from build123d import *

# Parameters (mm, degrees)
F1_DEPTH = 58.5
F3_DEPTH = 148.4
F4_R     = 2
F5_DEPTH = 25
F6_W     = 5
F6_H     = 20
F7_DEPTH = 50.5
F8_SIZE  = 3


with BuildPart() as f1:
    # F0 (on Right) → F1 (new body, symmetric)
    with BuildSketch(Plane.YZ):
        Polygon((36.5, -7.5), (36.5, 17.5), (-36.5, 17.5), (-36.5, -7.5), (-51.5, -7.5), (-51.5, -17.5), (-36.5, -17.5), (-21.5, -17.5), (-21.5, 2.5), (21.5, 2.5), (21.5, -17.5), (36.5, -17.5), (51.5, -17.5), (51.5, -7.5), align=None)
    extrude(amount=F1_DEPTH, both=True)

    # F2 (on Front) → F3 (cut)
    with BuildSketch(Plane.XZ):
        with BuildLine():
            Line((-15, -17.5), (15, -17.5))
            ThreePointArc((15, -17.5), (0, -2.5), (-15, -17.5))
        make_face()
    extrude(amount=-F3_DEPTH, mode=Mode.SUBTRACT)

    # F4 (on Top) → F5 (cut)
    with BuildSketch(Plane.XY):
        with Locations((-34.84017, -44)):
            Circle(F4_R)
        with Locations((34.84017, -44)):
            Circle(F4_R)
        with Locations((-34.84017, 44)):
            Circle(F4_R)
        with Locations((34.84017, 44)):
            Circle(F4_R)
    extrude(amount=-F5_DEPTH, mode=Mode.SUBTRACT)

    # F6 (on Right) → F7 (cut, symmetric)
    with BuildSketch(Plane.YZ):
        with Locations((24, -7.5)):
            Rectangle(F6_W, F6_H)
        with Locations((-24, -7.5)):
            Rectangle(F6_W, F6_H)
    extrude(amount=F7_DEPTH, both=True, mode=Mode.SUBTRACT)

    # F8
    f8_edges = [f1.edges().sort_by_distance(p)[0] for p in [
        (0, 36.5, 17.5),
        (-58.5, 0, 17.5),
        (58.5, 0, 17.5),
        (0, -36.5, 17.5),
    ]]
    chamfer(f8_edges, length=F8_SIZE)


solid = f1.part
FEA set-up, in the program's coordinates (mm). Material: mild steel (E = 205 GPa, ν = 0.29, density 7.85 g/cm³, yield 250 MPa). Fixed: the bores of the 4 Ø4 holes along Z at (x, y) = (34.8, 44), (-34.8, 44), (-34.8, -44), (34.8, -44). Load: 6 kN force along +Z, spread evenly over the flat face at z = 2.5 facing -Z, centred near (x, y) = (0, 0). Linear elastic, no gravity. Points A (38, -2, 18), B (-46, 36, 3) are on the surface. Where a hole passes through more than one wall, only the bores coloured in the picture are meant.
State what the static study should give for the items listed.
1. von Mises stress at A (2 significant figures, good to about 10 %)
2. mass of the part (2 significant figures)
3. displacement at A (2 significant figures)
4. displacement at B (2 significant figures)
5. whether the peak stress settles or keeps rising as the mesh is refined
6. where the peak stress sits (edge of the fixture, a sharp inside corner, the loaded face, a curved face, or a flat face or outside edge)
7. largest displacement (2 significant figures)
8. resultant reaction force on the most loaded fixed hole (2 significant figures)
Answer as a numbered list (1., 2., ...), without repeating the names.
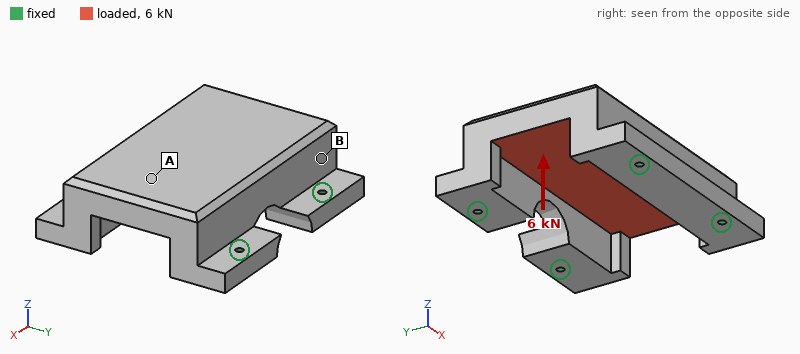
1. 6.9 MPa
2. 1.6 kg
3. 3.6 µm
4. 1.8 µm
5. keeps rising
6. edge of the fixture
7. 4.0 µm
8. 1.9 kN
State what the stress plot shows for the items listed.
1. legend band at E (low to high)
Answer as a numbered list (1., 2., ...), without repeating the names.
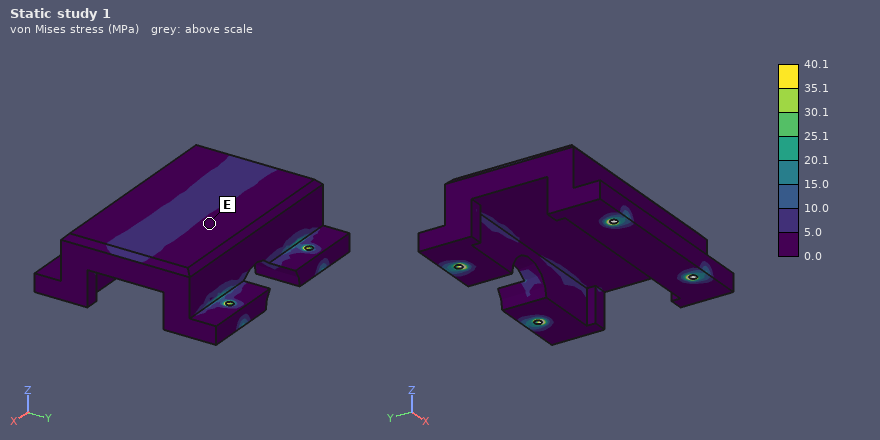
1. 0.0 to 5.0 MPa
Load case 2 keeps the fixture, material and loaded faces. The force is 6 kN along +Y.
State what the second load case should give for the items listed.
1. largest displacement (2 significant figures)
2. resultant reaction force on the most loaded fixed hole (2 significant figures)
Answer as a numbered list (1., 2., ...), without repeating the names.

1. 3.9 µm
2. 1.6 kN
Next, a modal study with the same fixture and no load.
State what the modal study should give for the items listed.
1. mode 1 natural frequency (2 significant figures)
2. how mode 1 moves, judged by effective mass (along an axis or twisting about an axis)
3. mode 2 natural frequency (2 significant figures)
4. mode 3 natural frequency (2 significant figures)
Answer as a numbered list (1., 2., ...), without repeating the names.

1. 5400 Hz
2. along X
3. 6400 Hz
4. 6500 Hz
